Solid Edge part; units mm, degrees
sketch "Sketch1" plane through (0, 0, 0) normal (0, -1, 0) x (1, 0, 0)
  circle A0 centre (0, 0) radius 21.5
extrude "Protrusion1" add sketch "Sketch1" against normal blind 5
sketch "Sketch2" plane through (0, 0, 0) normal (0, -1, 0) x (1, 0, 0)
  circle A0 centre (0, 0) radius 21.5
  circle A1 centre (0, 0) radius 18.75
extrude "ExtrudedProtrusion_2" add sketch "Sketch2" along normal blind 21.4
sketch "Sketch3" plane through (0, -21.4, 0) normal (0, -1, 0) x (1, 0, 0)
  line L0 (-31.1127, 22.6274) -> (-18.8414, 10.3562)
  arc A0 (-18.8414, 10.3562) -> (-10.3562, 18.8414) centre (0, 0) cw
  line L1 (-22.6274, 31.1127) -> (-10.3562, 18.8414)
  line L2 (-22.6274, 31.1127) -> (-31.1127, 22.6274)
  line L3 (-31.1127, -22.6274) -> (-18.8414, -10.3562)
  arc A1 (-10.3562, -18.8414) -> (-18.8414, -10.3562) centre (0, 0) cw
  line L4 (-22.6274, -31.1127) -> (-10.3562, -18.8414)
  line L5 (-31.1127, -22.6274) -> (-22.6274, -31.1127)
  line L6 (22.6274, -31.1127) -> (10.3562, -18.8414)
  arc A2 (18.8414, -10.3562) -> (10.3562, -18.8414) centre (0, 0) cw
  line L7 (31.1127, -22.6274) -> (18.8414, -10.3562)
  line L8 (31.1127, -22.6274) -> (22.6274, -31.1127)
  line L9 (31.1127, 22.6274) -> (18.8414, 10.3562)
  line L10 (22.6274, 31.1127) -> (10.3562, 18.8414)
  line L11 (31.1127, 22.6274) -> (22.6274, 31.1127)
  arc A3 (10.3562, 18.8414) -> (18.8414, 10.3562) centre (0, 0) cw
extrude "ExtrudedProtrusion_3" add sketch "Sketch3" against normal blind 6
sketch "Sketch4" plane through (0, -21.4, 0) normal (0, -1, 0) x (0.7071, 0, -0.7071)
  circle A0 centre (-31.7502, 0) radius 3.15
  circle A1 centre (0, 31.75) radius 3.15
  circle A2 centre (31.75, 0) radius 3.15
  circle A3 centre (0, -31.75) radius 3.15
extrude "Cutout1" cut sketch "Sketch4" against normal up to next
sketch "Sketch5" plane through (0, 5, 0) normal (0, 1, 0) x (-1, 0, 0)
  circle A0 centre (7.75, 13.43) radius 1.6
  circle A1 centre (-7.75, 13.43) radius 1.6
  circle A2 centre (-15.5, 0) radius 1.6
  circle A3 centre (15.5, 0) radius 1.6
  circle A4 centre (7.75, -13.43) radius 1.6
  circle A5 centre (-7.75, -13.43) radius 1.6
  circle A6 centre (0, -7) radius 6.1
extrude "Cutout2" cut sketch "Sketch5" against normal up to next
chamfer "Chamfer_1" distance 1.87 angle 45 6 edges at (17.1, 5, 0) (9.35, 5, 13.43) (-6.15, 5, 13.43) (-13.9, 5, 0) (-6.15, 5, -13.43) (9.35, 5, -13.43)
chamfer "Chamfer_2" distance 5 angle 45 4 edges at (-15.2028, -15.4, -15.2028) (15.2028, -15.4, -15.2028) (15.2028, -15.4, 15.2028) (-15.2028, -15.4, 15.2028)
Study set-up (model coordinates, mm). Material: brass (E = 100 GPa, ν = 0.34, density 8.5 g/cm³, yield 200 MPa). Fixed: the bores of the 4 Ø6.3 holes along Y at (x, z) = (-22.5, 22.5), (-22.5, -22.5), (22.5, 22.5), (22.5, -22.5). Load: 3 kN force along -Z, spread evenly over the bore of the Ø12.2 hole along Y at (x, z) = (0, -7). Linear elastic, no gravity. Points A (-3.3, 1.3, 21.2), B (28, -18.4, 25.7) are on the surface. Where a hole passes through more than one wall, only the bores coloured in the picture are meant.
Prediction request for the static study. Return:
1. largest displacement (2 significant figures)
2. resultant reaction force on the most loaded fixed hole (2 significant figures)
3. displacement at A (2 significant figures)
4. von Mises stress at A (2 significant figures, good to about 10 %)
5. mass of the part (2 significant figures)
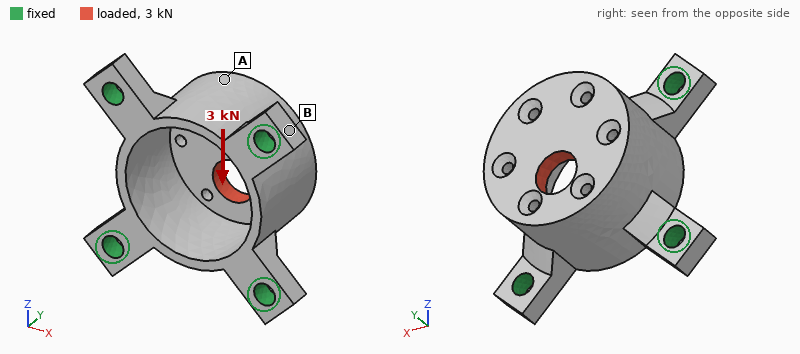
26 µm
1.1 kN
20 µm
14 MPa
160 g
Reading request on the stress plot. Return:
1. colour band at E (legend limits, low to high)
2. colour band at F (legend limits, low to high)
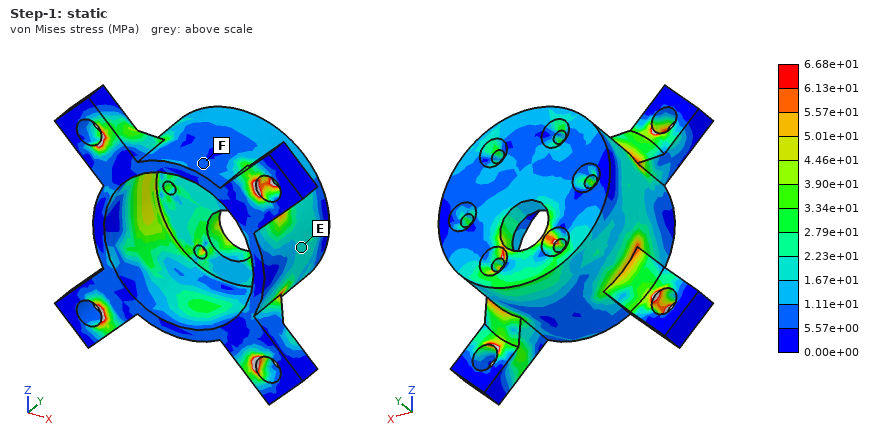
1.67e+01 to 2.23e+01 MPa
5.57e+00 to 1.11e+01 MPa
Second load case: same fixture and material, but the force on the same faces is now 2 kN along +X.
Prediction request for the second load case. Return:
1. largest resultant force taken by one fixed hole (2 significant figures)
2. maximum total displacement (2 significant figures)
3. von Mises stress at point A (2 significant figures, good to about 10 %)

810 N
16 µm
6.2 MPa
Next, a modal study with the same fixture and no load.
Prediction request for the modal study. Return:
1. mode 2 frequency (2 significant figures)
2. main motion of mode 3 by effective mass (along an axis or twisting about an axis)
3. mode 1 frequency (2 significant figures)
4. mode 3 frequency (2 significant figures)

7200 Hz
along Y
7200 Hz
8600 Hz
